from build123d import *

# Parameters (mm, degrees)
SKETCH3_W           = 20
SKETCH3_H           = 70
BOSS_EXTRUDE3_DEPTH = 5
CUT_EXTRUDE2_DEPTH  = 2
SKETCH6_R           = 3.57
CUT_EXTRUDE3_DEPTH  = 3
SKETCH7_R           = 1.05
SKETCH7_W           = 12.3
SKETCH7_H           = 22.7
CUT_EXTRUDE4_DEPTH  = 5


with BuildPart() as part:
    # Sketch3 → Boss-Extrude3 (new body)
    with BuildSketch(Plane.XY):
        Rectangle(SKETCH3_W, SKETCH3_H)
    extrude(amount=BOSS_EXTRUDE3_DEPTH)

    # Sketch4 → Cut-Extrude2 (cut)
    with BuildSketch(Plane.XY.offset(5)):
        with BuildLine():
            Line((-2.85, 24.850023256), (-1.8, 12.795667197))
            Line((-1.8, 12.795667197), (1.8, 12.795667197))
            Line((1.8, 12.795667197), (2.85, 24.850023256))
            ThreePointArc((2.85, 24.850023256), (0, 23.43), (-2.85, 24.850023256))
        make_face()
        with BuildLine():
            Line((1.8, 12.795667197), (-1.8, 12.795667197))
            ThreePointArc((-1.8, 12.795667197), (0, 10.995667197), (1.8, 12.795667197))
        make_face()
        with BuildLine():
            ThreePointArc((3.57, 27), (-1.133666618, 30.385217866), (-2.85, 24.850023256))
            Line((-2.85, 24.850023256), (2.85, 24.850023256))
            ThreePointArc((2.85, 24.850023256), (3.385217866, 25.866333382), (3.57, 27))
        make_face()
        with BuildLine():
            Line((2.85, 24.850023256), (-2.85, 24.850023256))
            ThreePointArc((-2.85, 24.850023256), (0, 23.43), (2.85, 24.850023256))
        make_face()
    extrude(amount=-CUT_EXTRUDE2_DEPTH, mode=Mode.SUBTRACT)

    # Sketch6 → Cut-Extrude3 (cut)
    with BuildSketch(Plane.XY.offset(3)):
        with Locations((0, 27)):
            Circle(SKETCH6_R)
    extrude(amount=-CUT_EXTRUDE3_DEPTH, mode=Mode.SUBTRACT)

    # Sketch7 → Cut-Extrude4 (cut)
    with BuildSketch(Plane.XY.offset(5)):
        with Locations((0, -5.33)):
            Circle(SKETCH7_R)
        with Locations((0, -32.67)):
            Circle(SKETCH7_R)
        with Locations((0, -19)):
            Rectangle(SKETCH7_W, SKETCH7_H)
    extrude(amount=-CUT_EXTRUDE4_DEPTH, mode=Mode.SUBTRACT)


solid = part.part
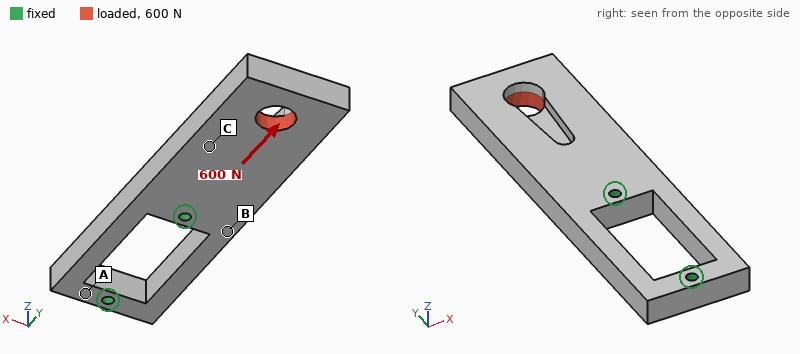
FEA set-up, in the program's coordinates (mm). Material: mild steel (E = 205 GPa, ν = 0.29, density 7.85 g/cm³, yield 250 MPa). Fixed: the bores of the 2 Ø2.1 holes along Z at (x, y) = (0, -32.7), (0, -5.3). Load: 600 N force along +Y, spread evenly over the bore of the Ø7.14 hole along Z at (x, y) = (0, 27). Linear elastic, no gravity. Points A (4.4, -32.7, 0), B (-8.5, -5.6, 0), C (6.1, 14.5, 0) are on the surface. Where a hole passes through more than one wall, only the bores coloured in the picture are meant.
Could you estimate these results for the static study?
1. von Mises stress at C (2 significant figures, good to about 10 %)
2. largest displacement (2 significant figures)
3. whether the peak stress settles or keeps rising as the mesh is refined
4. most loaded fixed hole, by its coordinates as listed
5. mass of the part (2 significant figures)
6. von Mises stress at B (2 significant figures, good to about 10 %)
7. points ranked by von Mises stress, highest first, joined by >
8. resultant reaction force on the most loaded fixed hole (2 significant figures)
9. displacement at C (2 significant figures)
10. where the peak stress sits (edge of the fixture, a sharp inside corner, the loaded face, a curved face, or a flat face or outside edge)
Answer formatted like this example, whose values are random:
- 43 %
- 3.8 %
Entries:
- 13 MPa
- 13 µm
- keeps rising
- (0, -5.3)
- 41 g
- 6.0 MPa
- C > B > A
- 550 N
- 3.9 µm
- edge of the fixture
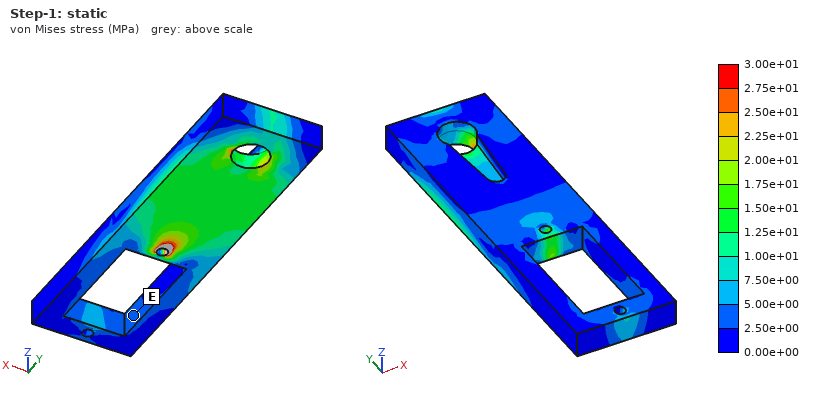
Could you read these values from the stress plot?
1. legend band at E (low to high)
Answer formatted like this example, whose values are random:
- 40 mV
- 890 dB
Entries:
- 2.50e+00 to 5.00e+00 MPa
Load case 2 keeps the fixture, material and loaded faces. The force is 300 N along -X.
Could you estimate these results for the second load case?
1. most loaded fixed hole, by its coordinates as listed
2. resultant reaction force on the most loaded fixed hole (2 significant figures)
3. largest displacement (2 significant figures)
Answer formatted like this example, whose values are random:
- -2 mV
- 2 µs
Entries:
- (0, -5.3)
- 410 N
- 41 µm
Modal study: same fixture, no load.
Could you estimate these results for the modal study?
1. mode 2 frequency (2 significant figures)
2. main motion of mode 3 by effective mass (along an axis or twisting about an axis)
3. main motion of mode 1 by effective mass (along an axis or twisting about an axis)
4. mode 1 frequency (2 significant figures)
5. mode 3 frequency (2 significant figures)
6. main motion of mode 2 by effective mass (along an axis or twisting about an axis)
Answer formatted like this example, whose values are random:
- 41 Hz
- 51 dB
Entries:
- 4000 Hz
- twisting about Y
- along Z
- 2400 Hz
- 7600 Hz
- along X
